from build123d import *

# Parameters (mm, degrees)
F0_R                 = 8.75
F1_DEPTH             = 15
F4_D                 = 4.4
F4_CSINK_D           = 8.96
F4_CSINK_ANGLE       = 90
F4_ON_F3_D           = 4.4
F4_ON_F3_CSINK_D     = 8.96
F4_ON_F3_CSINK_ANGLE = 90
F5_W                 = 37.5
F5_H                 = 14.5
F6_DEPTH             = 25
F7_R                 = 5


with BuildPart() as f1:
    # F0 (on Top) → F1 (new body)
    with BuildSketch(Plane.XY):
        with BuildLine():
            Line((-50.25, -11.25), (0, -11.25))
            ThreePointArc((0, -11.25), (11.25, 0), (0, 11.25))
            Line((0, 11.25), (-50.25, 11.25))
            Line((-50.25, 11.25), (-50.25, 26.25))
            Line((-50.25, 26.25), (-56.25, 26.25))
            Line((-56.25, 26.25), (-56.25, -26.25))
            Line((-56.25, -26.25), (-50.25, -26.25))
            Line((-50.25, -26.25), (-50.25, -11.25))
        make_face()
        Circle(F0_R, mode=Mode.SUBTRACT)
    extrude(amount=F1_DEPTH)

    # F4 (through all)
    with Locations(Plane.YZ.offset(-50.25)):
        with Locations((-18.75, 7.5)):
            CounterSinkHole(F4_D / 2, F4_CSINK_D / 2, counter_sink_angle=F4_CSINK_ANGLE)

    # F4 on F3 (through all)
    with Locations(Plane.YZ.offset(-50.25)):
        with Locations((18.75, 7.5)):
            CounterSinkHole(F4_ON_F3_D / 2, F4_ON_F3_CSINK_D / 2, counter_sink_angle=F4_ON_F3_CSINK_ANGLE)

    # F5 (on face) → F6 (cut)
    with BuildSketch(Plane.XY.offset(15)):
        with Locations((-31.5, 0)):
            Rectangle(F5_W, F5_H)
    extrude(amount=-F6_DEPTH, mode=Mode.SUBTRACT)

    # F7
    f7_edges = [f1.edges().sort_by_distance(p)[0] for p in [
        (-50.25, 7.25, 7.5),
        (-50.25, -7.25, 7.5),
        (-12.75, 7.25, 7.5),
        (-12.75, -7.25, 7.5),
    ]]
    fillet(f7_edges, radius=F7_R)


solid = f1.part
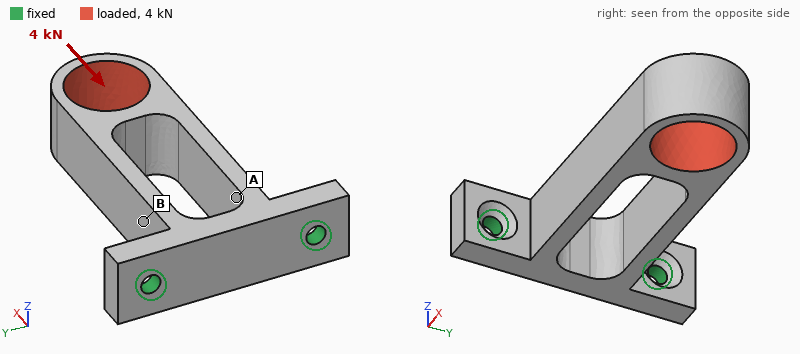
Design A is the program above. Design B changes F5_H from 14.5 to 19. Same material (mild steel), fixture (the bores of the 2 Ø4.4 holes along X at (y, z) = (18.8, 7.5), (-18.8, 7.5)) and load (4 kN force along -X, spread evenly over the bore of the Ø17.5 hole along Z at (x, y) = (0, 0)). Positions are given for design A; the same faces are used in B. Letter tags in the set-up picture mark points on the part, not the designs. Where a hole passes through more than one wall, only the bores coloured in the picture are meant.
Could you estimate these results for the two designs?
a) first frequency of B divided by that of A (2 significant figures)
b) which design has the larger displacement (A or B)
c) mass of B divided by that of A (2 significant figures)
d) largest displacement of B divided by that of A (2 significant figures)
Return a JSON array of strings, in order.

["0.53", "B", "0.80", "1.2"]
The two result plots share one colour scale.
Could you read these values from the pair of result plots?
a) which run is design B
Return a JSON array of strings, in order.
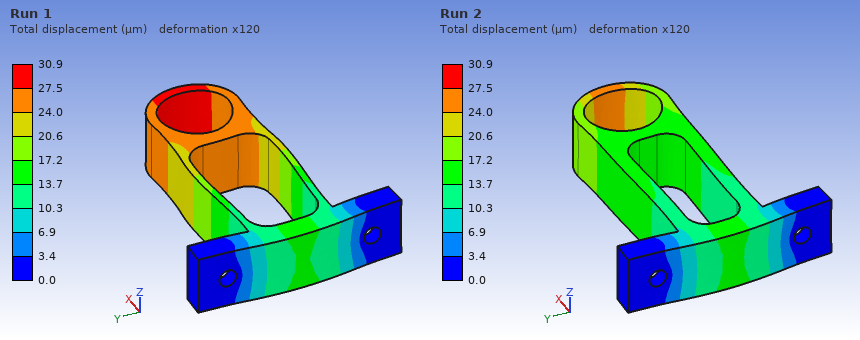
["Run 1"]
